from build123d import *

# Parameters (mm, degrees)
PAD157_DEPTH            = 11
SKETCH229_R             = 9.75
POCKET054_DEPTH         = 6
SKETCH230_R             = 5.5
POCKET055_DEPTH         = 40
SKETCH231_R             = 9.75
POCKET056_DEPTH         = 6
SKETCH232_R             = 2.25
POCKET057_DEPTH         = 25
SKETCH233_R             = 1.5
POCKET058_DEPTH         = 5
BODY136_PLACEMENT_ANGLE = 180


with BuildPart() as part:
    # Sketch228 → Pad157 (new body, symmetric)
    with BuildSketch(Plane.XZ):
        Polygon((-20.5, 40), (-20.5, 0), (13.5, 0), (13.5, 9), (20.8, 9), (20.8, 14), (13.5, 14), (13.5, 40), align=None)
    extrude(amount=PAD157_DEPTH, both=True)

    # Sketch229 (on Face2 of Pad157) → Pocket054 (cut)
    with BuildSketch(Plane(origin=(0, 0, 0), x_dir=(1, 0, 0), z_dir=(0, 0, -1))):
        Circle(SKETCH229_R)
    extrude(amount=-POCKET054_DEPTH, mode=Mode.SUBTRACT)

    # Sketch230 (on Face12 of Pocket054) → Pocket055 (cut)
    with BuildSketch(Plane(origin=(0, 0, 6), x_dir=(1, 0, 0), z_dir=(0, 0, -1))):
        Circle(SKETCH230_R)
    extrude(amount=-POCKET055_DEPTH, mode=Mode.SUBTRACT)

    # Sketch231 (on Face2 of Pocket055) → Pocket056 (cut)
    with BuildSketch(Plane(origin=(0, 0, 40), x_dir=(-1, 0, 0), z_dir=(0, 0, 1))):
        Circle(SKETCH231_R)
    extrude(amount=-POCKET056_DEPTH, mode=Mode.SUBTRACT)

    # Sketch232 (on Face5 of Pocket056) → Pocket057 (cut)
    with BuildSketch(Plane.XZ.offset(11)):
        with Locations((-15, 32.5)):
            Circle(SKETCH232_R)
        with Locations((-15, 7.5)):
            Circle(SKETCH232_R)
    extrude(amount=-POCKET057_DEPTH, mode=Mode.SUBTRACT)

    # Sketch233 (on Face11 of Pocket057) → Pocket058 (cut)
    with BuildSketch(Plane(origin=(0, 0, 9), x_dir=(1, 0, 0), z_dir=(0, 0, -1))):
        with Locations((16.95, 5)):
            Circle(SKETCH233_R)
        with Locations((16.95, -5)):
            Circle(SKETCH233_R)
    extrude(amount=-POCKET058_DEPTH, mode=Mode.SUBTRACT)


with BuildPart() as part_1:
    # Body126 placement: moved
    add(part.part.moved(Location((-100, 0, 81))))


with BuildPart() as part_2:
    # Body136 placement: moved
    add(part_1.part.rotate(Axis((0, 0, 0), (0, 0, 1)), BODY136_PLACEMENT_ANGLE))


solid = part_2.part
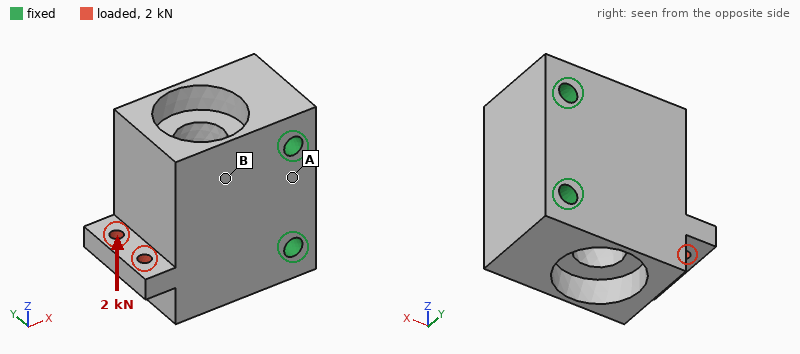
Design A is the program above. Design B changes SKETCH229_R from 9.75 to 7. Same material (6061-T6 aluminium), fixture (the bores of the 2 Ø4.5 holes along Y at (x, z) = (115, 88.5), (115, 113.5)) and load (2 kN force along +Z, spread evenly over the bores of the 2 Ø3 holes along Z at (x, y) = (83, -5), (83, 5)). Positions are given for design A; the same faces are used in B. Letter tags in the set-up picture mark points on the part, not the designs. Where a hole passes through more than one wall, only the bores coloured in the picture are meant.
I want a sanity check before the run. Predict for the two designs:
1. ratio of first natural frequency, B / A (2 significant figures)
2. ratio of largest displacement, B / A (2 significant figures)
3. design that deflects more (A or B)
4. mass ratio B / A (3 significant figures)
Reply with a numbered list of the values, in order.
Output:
1. 1.0
2. 0.92
3. A
4. 1.04
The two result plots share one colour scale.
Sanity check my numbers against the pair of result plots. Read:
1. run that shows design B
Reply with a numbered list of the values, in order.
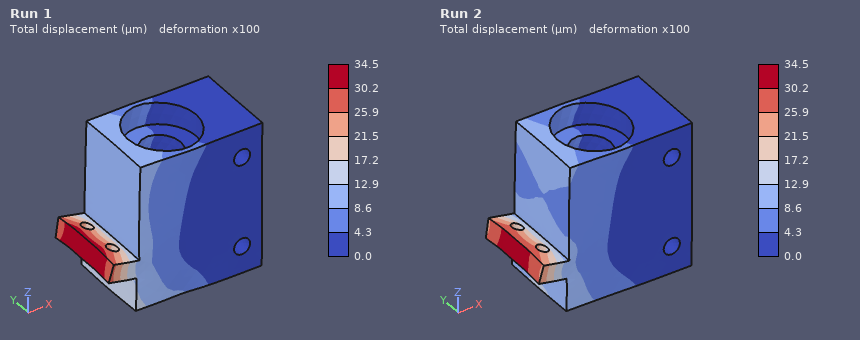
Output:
1. Run 2
